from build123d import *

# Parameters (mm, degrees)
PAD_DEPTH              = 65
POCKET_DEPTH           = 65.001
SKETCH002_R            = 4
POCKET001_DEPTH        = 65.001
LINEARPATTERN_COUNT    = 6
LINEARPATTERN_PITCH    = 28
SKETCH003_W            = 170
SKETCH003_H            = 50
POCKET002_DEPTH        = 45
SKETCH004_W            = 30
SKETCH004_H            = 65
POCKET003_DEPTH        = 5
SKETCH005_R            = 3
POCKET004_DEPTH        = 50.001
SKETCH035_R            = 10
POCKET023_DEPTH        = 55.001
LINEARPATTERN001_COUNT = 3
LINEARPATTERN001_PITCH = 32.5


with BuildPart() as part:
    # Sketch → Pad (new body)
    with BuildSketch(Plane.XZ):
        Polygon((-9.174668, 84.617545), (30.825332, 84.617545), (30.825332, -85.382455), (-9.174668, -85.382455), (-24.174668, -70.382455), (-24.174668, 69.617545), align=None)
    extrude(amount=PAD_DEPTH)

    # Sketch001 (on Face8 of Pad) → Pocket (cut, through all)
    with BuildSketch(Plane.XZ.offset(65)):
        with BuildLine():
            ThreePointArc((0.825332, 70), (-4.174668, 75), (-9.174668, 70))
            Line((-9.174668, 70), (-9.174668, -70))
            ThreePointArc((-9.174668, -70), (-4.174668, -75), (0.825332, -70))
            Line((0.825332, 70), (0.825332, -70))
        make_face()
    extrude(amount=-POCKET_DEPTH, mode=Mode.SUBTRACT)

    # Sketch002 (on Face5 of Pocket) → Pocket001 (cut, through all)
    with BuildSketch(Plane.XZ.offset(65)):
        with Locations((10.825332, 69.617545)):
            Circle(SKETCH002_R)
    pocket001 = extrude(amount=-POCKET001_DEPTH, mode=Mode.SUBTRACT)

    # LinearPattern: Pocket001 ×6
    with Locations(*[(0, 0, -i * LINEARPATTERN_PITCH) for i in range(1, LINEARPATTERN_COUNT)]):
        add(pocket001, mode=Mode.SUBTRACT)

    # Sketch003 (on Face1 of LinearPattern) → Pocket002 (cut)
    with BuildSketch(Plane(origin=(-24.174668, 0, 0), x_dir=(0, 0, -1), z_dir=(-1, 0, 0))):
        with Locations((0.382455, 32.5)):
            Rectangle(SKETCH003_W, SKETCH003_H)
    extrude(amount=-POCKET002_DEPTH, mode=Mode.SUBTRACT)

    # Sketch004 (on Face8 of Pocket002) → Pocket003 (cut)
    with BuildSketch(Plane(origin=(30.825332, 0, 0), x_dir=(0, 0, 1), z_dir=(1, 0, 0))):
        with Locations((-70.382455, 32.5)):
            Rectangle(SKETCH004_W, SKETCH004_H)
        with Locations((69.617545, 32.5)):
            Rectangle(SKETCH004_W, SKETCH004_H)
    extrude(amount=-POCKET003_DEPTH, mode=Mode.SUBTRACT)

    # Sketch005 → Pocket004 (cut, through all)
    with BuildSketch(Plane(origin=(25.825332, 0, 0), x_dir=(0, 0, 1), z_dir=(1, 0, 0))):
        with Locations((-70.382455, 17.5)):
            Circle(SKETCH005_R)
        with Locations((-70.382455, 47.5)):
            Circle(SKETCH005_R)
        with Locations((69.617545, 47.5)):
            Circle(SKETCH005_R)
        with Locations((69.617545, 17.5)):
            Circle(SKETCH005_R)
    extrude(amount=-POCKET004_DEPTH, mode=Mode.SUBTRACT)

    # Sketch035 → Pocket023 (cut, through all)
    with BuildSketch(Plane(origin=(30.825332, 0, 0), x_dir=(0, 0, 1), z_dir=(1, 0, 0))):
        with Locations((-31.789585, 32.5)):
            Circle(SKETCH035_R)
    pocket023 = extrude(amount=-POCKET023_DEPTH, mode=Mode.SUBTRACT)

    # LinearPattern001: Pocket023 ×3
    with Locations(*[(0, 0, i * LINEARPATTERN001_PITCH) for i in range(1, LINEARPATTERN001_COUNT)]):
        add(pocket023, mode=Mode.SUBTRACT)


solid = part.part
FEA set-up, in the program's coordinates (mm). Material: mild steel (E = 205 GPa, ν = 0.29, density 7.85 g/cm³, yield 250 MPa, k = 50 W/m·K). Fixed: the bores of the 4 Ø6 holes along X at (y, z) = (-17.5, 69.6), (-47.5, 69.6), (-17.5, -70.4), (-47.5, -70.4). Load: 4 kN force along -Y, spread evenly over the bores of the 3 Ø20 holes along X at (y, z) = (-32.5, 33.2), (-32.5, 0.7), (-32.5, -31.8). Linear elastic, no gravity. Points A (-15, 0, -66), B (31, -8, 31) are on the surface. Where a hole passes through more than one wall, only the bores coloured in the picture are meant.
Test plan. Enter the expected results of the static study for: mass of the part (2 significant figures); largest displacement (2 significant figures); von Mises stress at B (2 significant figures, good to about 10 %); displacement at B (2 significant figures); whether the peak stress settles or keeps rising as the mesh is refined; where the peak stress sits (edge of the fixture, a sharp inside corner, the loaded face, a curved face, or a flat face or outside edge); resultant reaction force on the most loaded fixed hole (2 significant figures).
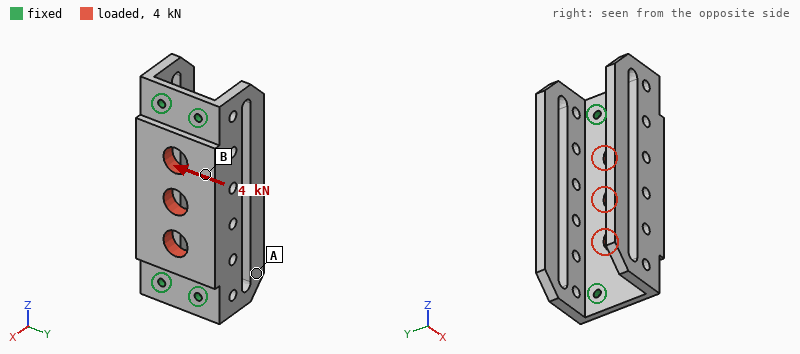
1.3 kg
6.5 µm
5.6 MPa
4.2 µm
keeps rising
edge of the fixture
1.2 kN
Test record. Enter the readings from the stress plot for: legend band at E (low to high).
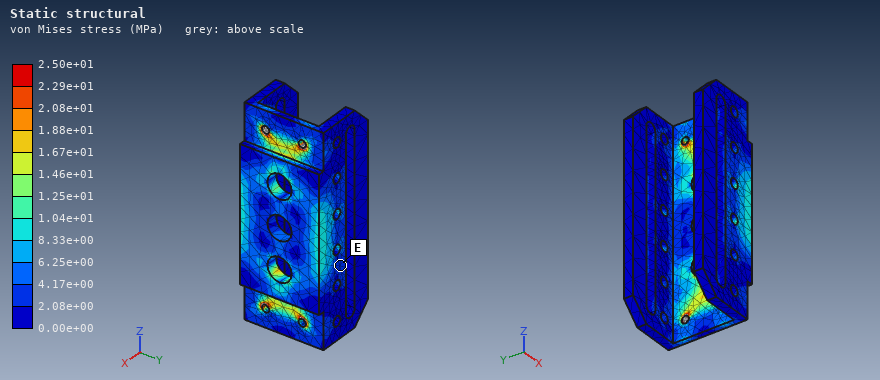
2.08e+00 to 4.17e+00 MPa
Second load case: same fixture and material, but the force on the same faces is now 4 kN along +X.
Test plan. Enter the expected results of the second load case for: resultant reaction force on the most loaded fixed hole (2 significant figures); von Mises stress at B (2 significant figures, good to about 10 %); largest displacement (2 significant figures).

1.1 kN
15 MPa
26 µm
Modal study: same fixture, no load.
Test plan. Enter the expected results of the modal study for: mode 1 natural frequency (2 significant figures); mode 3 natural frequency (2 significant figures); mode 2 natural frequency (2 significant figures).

820 Hz
1900 Hz
840 Hz
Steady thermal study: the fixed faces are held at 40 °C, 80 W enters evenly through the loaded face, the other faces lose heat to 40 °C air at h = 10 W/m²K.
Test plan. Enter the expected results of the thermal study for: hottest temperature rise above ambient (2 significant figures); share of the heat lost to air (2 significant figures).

69 K
20 %
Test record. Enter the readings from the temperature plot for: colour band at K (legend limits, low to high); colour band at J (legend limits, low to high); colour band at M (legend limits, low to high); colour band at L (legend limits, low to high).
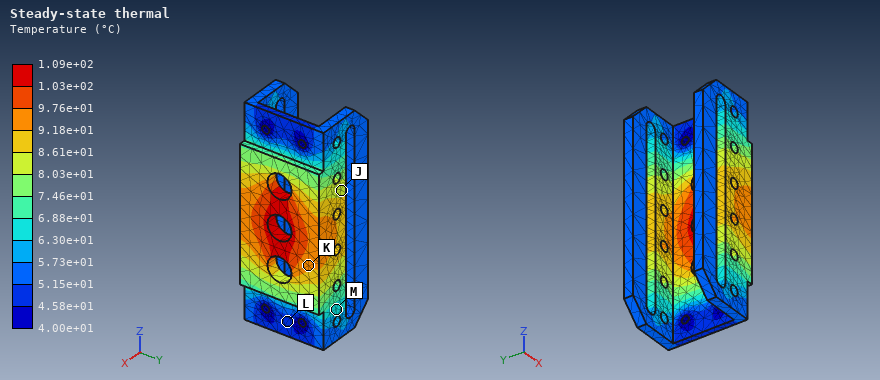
9.18e+01 to 9.76e+01 °C
8.03e+01 to 8.61e+01 °C
6.30e+01 to 6.88e+01 °C
4.58e+01 to 5.15e+01 °C
